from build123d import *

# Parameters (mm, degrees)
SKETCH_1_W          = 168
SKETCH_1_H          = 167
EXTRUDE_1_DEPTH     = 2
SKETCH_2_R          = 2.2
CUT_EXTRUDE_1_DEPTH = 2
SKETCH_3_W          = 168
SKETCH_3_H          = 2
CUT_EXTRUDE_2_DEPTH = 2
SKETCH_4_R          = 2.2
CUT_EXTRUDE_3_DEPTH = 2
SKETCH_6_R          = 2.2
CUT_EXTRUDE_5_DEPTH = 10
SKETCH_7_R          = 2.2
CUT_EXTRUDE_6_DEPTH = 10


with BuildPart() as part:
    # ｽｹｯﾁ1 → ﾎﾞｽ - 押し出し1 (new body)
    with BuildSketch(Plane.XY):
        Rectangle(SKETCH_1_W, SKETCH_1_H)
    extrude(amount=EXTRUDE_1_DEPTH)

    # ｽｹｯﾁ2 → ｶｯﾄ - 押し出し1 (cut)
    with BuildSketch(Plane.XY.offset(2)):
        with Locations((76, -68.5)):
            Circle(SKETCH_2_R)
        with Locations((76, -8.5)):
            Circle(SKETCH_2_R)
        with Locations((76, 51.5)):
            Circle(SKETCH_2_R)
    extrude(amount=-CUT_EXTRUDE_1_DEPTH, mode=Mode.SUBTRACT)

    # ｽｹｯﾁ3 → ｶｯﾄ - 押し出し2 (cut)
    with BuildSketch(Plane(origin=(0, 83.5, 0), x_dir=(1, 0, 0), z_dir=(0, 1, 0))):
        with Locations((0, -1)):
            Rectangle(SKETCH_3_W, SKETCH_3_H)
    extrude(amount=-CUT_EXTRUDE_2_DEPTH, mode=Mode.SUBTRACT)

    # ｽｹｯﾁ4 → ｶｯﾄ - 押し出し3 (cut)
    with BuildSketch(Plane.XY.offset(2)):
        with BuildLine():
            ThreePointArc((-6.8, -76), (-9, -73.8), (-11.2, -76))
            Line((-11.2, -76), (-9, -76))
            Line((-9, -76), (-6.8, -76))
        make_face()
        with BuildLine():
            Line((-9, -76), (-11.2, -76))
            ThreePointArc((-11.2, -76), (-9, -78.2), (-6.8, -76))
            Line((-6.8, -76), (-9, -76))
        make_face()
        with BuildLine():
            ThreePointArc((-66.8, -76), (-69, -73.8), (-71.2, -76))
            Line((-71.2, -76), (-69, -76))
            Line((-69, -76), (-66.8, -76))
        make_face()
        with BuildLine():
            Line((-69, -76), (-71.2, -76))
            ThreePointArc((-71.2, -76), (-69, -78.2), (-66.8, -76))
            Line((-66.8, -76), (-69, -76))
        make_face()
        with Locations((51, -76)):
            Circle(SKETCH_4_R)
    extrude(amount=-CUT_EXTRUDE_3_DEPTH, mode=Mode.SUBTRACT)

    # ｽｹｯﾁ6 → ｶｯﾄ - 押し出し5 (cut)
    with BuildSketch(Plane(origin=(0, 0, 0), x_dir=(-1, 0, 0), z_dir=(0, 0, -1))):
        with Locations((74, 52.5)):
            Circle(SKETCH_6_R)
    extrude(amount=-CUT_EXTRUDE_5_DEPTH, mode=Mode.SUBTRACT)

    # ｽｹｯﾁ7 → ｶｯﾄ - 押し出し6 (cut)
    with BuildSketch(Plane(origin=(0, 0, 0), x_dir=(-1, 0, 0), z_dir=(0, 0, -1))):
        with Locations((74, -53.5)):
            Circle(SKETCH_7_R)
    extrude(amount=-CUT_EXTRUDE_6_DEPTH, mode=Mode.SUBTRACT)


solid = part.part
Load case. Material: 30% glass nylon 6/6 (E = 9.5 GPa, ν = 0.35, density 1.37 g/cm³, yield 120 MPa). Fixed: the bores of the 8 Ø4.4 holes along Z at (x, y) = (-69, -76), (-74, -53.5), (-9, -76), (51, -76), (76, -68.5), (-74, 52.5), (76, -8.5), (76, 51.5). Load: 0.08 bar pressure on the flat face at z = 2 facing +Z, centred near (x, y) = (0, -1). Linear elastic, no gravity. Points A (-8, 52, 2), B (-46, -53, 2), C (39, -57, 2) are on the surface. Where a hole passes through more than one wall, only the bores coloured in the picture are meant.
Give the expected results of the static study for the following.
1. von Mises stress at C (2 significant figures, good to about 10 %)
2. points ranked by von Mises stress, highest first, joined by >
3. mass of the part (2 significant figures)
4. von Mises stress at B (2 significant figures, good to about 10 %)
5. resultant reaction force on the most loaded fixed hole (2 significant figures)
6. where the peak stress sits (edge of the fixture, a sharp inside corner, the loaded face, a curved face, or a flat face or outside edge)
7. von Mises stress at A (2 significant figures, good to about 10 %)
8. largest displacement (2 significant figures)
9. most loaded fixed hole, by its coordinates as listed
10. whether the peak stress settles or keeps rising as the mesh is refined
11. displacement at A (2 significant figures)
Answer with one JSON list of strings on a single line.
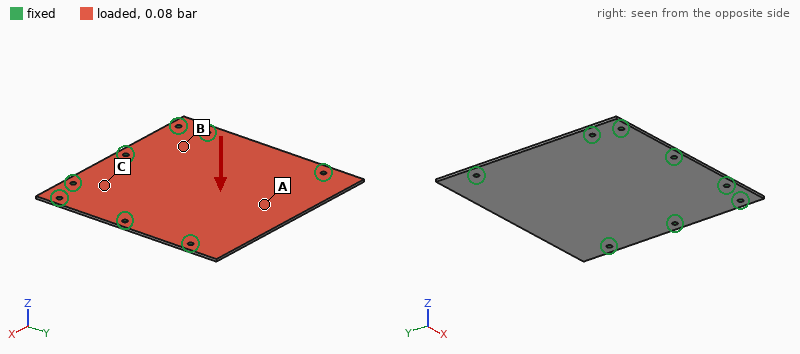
["3.4 MPa", "A > B > C", "76 g", "6.7 MPa", "55 N", "edge of the fixture", "11 MPa", "2.3 mm", "(-74, 52.5)", "keeps rising", "2.0 mm"]
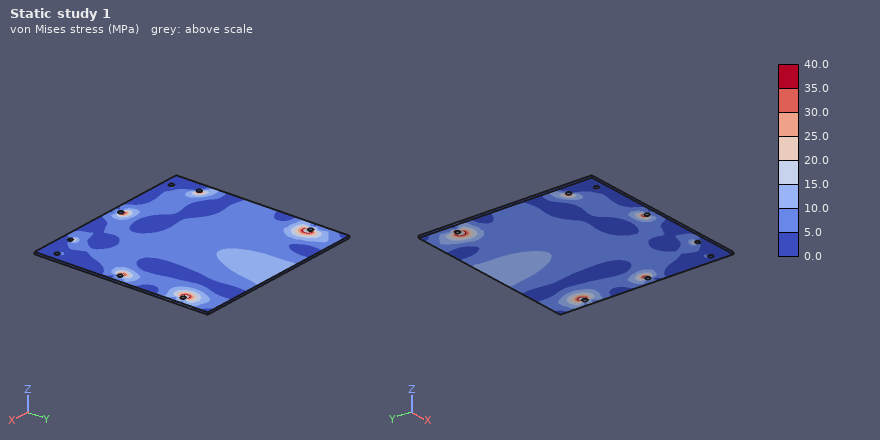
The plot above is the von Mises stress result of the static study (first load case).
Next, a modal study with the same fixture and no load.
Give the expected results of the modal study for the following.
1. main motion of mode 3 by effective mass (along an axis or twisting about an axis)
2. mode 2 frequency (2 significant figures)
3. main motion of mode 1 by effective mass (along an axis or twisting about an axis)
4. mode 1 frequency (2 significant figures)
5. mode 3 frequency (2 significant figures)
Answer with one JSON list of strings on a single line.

["twisting about Y", "340 Hz", "along Z", "230 Hz", "530 Hz"]
